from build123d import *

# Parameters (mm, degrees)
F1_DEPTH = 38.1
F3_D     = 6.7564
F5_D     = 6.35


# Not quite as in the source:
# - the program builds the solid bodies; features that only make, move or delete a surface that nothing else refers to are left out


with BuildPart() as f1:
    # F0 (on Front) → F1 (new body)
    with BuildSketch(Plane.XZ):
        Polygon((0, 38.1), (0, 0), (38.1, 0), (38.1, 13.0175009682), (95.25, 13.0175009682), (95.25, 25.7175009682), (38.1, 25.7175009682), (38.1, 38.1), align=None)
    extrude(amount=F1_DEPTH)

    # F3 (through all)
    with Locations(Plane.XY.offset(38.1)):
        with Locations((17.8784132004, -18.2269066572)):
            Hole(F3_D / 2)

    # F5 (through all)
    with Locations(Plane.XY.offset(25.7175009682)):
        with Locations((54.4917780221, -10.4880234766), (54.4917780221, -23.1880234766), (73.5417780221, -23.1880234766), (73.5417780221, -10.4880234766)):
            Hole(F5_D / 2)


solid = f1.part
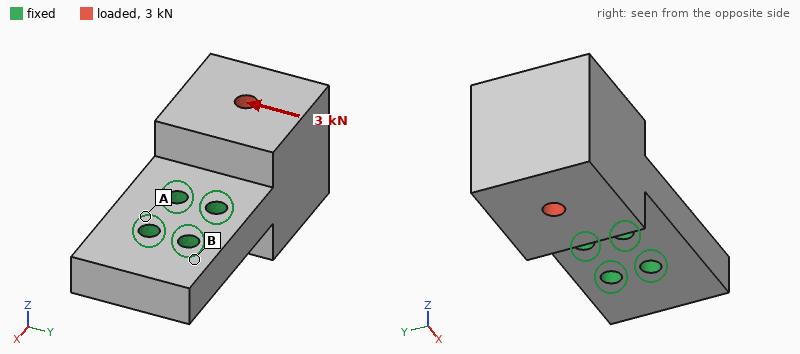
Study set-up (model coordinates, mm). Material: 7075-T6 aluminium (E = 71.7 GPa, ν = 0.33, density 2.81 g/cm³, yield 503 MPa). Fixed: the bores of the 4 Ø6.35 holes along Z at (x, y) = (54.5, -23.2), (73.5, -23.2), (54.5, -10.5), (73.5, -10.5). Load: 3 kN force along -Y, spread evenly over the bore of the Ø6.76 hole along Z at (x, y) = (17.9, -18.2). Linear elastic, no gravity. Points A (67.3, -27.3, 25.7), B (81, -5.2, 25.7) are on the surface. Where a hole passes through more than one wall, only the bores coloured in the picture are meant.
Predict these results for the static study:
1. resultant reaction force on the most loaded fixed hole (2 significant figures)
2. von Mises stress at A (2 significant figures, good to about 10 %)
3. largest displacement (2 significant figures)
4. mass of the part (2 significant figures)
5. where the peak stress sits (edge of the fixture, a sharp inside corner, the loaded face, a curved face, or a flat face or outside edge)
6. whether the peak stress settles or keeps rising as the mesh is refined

4.4 kN
11 MPa
37 µm
220 g
edge of the fixture
keeps rising
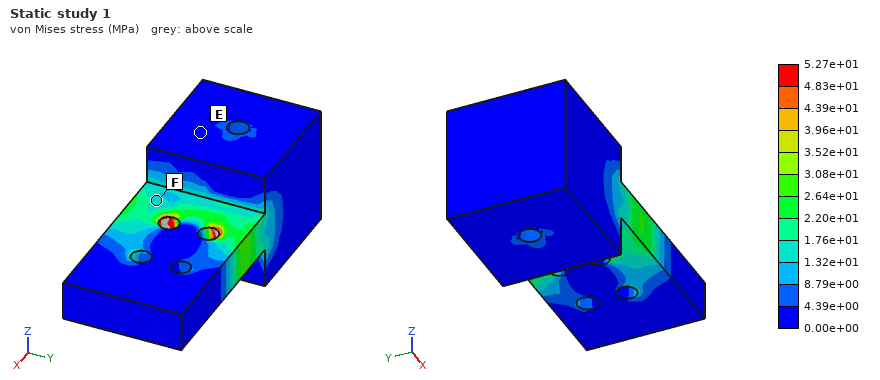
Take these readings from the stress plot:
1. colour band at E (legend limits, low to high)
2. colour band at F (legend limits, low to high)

0.00e+00 to 4.39e+00 MPa
1.32e+01 to 1.76e+01 MPa
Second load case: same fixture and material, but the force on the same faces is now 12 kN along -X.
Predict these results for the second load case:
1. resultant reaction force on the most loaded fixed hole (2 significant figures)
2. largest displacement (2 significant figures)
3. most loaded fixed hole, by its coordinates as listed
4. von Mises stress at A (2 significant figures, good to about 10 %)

5.7 kN
16 µm
(54.5, -23.2)
7.2 MPa
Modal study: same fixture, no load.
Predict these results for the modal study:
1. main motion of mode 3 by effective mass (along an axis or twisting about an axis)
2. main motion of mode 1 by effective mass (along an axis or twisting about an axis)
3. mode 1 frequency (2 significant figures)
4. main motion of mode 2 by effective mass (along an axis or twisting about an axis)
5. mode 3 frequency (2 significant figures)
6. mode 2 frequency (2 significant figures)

twisting about X
along Z
2100 Hz
along Y
5700 Hz
4400 Hz
